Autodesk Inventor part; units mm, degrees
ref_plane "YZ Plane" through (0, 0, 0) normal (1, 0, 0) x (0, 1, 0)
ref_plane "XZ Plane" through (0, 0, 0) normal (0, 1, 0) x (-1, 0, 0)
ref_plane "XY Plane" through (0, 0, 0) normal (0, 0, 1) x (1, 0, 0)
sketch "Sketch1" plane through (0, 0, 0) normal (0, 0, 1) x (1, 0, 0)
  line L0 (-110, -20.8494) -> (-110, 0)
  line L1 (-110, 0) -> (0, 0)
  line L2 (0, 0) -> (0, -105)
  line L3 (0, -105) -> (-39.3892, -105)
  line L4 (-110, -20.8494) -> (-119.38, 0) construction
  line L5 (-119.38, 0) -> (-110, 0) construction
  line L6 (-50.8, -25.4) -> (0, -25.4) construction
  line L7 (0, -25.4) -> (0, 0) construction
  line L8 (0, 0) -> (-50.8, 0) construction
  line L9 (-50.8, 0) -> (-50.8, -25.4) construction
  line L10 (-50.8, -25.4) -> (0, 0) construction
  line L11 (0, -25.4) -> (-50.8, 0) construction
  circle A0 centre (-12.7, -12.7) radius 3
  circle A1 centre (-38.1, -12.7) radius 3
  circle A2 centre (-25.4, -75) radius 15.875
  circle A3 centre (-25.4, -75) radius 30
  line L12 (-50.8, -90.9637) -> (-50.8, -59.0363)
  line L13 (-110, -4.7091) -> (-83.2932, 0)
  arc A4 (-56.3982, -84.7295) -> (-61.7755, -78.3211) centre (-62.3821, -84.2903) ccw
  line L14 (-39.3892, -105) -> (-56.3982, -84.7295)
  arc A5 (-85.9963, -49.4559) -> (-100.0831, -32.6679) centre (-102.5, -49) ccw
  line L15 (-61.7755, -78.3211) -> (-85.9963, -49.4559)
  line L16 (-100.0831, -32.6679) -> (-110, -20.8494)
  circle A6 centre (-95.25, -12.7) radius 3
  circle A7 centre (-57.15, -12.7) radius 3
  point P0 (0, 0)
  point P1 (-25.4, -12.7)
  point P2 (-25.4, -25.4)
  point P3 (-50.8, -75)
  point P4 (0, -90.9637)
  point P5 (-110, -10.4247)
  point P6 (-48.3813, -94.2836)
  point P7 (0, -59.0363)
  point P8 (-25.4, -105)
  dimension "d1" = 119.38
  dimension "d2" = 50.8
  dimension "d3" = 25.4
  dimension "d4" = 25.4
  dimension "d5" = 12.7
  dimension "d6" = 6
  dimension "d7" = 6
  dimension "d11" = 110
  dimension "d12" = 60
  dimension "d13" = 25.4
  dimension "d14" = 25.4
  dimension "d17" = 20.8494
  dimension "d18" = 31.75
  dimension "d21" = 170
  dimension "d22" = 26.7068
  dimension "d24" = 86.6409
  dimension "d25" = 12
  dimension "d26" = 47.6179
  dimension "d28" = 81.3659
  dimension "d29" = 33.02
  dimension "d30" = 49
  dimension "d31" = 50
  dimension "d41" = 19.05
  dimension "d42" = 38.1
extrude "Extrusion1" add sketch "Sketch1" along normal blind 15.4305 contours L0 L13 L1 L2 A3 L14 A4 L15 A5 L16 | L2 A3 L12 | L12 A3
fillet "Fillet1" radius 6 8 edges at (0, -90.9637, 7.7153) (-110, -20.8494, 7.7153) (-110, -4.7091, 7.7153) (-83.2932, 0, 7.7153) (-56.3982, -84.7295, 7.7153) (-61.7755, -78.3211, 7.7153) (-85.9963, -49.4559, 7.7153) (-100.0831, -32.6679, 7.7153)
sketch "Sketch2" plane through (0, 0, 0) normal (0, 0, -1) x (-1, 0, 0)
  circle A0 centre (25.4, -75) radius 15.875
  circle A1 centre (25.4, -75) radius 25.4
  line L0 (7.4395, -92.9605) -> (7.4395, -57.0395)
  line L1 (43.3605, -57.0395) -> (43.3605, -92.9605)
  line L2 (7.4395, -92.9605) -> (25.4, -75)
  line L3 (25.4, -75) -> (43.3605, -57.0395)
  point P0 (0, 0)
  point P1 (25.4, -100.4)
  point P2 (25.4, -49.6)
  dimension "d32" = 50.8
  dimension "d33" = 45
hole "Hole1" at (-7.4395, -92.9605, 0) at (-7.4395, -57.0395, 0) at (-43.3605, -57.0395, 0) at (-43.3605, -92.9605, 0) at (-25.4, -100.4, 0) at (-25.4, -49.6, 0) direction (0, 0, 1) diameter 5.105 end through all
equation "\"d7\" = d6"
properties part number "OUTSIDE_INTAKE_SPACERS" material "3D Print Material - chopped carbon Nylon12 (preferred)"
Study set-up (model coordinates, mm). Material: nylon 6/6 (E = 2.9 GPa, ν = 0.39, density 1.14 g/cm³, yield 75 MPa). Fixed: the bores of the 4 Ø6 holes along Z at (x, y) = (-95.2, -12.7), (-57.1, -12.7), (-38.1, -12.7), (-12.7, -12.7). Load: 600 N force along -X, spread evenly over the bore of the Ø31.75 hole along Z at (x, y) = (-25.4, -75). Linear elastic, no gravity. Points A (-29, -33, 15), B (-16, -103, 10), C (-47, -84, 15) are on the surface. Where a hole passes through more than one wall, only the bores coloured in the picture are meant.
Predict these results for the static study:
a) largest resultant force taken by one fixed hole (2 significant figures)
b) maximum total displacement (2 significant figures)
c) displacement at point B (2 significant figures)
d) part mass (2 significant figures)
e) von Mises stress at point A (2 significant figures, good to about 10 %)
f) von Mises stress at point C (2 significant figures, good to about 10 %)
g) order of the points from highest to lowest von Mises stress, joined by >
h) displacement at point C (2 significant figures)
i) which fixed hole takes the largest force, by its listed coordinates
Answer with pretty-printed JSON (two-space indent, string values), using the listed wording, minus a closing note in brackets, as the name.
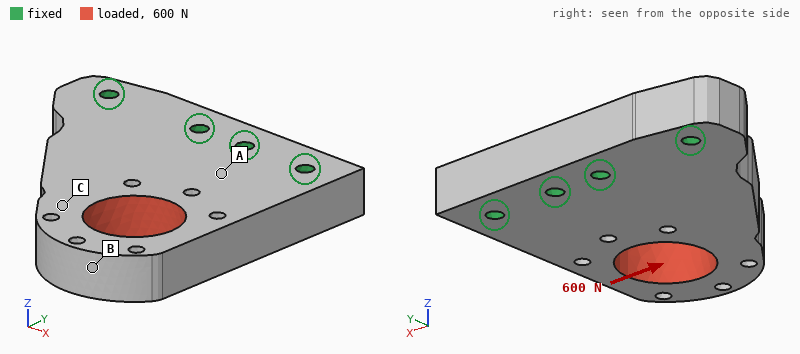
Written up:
{
  "largest resultant force taken by one fixed hole": "490 N",
  "maximum total displacement": "0.11 mm",
  "displacement at point B": "0.10 mm",
  "part mass": "130 g",
  "von Mises stress at point A": "1.2 MPa",
  "von Mises stress at point C": "1.9 MPa",
  "order of the points from highest to lowest von Mises stress, joined by >": "C > A > B",
  "displacement at point C": "0.073 mm",
  "which fixed hole takes the largest force, by its listed coordinates": "(-12.7, -12.7)"
}
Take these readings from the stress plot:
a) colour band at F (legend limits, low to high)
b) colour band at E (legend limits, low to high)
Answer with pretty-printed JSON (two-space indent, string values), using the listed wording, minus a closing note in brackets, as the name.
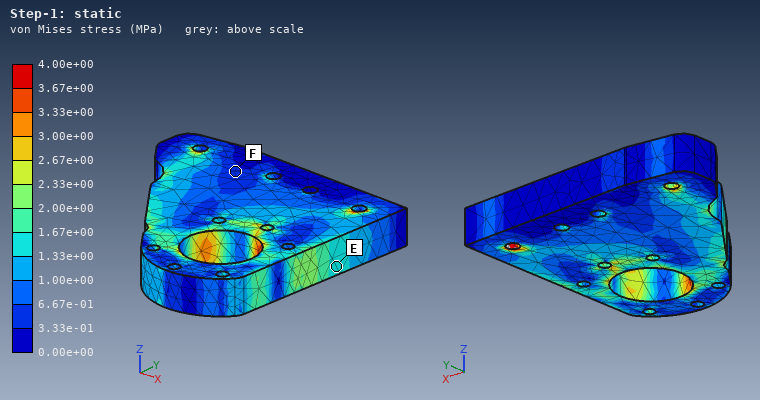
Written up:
{
  "colour band at F": "3.33e-01 to 6.67e-01 MPa",
  "colour band at E": "1.33e+00 to 1.67e+00 MPa"
}
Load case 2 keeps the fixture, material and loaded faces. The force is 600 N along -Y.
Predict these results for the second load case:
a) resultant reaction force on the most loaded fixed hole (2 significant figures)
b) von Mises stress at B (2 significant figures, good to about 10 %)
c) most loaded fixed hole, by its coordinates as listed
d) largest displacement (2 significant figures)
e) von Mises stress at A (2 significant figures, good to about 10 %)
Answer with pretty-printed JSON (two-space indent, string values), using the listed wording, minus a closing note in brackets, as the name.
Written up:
{
  "resultant reaction force on the most loaded fixed hole": "360 N",
  "von Mises stress at B": "0.90 MPa",
  "most loaded fixed hole, by its coordinates as listed": "(-12.7, -12.7)",
  "largest displacement": "47 µm",
  "von Mises stress at A": "0.52 MPa"
}
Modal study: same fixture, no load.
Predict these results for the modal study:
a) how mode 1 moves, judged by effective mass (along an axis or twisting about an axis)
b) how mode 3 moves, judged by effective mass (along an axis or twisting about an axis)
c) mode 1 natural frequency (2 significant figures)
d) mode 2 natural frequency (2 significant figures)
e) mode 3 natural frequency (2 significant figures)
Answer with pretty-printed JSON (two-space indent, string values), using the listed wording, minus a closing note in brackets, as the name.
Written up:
{
  "how mode 1 moves, judged by effective mass": "along Z",
  "how mode 3 moves, judged by effective mass": "along X",
  "mode 1 natural frequency": "670 Hz",
  "mode 2 natural frequency": "1600 Hz",
  "mode 3 natural frequency": "2200 Hz"
}
